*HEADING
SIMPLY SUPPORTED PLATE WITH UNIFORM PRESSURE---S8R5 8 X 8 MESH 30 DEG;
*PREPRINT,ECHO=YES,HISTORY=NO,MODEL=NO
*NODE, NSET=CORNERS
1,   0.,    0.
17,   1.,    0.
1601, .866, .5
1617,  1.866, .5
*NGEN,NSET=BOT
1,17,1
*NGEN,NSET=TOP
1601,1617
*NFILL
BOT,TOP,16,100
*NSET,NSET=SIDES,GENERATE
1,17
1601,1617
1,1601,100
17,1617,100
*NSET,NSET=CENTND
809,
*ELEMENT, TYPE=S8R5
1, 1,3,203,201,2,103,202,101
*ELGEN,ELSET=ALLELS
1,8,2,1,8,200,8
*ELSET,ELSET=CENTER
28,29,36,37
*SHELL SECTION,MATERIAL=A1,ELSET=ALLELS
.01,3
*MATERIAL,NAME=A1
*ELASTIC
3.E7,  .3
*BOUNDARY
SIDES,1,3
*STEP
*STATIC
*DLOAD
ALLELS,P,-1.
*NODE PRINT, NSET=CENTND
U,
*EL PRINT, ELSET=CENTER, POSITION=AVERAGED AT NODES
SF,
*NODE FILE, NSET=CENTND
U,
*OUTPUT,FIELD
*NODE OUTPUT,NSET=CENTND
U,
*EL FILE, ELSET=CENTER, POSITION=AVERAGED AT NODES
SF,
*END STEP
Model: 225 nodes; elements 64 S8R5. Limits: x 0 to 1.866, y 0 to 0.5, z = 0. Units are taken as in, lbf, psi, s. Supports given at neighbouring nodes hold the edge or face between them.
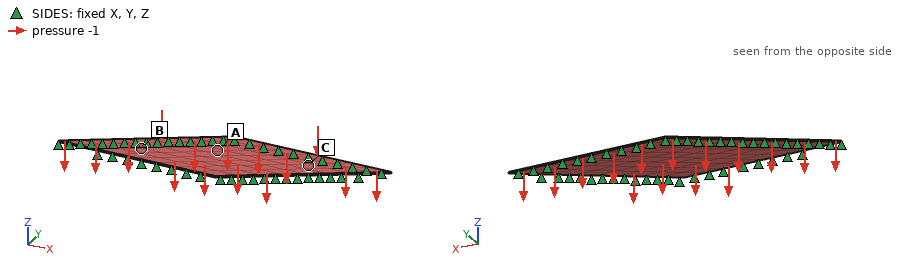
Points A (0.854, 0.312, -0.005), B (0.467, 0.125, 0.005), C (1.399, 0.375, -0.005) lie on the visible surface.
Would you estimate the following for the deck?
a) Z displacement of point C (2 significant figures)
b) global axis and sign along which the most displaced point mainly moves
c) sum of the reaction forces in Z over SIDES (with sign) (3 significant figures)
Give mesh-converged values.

-2.9e-05 in
-Z
0.500 lbf
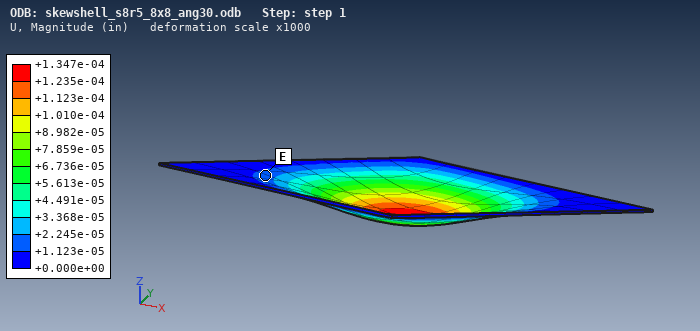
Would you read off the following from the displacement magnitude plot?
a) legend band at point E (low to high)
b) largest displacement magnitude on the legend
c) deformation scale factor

+1.123e-05 to +2.245e-05 in
+1.347e-04 in
1000
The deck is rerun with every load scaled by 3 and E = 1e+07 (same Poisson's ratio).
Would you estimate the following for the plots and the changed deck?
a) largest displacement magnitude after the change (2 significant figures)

0.0012 in
